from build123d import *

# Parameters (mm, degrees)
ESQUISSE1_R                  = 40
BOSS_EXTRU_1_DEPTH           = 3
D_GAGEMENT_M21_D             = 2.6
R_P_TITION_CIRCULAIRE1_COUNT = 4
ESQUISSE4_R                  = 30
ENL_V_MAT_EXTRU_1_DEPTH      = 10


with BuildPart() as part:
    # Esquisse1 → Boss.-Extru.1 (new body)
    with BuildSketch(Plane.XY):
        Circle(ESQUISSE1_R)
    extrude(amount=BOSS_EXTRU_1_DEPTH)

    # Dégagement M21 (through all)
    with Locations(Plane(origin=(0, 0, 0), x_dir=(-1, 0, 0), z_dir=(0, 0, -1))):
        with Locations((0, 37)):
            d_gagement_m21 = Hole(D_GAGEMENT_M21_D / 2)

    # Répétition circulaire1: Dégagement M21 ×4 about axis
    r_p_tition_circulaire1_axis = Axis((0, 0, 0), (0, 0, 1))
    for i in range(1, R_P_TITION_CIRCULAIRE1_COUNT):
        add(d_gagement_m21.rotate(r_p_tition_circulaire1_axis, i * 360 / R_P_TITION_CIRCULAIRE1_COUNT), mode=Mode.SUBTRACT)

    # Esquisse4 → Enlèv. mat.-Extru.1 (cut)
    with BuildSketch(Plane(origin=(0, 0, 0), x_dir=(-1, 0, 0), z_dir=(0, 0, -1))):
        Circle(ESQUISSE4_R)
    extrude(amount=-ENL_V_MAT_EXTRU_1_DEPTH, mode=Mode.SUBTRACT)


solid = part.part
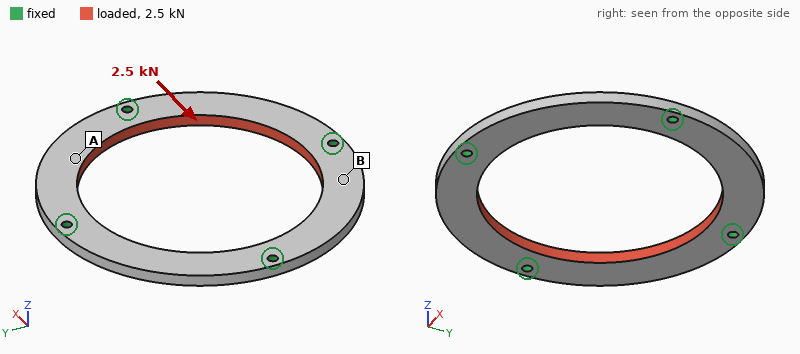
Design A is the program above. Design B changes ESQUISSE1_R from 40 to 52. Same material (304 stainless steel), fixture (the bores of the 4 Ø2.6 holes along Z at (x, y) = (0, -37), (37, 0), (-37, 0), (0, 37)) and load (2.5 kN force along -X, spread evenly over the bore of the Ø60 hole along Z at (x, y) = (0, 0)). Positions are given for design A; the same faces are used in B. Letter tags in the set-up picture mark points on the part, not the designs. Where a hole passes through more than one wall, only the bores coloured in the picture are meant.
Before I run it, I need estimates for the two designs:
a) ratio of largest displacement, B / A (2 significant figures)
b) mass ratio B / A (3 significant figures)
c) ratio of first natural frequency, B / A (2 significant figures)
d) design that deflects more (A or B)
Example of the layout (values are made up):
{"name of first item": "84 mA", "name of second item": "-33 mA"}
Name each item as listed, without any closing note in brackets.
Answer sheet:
{"ratio of largest displacement, B / A": "0.45", "mass ratio B / A": "2.59", "ratio of first natural frequency, B / A": "0.57", "design that deflects more": "A"}
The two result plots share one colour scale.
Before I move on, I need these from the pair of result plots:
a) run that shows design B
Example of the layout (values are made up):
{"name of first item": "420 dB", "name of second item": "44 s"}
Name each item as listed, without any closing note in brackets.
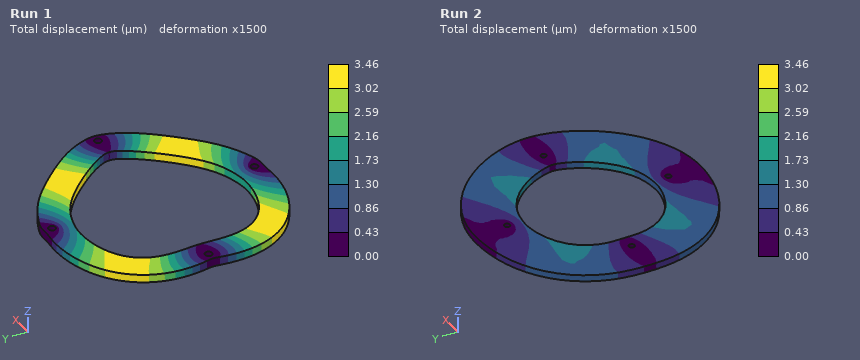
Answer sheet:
{"run that shows design B": "Run 2"}
